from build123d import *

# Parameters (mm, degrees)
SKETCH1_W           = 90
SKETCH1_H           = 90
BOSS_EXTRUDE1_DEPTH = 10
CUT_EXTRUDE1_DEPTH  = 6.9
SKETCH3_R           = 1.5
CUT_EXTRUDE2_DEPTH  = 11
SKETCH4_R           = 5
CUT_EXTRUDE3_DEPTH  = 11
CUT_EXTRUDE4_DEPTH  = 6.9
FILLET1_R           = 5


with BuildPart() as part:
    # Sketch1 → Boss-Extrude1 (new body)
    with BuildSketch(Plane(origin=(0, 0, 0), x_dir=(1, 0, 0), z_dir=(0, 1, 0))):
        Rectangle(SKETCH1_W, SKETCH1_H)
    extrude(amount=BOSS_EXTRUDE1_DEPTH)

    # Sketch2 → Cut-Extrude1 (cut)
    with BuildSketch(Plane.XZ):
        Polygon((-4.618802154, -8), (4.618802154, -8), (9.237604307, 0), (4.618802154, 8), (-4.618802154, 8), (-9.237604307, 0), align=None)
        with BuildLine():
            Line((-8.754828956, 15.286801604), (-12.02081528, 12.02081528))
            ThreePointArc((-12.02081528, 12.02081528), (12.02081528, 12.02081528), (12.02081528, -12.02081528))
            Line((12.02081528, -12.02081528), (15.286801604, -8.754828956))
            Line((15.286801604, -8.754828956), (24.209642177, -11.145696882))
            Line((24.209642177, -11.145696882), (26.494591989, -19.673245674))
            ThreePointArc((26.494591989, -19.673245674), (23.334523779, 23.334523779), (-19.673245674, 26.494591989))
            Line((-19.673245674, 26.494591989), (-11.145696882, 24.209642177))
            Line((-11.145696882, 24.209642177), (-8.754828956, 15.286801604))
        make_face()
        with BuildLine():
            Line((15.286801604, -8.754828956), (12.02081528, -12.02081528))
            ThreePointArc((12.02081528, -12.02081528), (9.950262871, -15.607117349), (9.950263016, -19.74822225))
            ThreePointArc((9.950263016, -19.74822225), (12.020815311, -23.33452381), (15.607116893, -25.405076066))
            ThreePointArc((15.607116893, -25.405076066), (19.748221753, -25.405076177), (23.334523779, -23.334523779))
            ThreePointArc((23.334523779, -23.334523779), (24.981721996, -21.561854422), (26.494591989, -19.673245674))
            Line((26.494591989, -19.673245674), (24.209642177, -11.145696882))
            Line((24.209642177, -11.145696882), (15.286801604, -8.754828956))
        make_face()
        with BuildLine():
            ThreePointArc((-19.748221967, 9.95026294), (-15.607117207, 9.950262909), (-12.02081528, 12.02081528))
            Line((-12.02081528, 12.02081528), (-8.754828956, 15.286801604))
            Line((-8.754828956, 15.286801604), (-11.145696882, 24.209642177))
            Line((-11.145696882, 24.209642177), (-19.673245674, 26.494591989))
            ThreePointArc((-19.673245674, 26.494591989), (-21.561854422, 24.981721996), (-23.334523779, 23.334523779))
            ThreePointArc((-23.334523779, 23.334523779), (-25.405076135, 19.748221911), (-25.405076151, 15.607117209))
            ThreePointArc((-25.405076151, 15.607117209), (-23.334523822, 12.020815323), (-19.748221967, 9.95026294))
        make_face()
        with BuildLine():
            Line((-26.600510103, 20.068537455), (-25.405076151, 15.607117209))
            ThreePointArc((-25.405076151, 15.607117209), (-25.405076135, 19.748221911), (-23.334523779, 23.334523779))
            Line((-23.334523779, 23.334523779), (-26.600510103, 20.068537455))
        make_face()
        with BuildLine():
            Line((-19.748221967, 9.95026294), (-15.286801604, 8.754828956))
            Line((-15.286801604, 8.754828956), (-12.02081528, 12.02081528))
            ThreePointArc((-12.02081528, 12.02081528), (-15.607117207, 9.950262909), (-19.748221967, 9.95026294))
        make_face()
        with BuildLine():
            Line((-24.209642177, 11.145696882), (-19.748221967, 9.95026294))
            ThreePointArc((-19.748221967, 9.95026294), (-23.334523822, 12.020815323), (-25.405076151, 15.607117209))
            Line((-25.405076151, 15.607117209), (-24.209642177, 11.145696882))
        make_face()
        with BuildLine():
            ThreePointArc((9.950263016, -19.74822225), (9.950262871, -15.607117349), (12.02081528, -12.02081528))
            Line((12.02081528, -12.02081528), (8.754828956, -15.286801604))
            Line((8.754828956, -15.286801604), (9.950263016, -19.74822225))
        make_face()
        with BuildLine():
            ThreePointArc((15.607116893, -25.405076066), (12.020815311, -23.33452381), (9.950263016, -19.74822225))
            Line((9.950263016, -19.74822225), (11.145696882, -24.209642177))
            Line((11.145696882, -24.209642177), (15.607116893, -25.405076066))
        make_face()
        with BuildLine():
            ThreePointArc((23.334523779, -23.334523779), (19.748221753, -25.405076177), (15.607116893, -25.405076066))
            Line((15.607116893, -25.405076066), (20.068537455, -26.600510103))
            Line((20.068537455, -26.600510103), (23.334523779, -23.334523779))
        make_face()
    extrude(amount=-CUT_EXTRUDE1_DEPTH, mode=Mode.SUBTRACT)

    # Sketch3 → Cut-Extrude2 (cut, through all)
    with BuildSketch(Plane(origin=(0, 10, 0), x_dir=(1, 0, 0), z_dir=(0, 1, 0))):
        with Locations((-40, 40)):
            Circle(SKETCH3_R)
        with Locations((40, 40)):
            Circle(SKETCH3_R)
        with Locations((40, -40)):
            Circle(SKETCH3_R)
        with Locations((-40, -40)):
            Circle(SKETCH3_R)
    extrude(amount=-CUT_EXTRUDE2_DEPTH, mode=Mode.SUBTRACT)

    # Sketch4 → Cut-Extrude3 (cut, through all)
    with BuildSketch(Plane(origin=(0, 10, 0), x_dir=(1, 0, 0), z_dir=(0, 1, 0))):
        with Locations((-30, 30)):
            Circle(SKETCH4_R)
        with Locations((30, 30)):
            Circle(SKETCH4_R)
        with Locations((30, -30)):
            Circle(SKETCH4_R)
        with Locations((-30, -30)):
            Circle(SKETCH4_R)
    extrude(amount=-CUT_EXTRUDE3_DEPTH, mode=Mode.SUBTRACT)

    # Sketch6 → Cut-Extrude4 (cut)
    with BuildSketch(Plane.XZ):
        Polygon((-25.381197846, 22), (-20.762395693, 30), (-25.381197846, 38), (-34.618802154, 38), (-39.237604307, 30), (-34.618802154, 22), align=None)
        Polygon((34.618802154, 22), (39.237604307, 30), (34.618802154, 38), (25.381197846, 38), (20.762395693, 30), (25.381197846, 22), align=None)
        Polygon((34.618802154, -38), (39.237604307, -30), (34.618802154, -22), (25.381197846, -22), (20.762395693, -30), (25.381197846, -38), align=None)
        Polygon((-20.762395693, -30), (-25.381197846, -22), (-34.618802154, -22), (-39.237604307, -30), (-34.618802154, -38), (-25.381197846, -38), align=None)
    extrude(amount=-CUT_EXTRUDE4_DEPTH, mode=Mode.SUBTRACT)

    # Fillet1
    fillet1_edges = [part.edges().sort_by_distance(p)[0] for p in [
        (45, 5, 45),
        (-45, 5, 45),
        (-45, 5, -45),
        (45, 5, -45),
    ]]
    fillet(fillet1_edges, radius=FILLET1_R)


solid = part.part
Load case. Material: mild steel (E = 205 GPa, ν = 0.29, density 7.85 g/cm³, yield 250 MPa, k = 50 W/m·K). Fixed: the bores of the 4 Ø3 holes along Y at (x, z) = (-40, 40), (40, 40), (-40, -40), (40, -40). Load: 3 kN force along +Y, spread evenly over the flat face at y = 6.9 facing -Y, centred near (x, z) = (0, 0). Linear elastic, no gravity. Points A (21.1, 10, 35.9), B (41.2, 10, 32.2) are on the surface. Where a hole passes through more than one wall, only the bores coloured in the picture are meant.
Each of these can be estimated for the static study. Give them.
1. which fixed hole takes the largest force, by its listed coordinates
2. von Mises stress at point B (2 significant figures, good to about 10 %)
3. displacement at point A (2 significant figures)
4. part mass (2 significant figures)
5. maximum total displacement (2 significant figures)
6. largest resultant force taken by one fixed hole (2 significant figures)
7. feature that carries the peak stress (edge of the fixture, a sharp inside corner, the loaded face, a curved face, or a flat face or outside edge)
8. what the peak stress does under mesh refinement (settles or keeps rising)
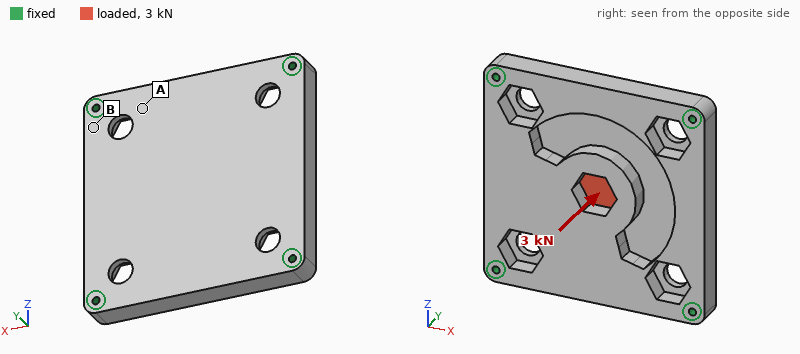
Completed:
(40, 40)
37 MPa
11 µm
480 g
48 µm
960 N
edge of the fixture
keeps rising
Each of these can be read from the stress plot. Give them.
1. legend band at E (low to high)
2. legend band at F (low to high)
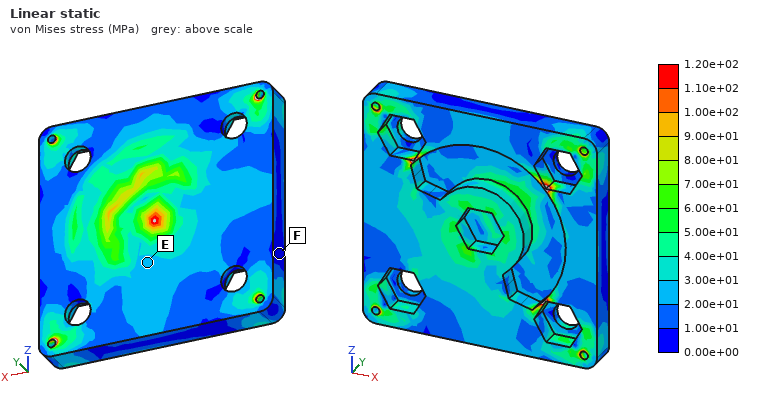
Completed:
2.00e+01 to 3.00e+01 MPa
0.00e+00 to 1.00e+01 MPa
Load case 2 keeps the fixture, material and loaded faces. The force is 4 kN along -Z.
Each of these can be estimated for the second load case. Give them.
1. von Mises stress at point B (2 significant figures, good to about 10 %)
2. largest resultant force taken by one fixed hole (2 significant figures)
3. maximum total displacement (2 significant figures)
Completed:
11 MPa
1.2 kN
5.4 µm
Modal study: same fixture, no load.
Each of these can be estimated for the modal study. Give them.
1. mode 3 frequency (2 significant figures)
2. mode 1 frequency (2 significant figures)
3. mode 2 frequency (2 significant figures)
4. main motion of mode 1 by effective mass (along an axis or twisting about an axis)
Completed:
6700 Hz
3700 Hz
6700 Hz
along Y
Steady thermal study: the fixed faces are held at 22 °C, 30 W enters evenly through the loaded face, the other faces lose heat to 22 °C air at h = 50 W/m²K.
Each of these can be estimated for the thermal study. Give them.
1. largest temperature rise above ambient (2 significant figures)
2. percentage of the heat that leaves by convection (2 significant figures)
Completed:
53 K
47 %
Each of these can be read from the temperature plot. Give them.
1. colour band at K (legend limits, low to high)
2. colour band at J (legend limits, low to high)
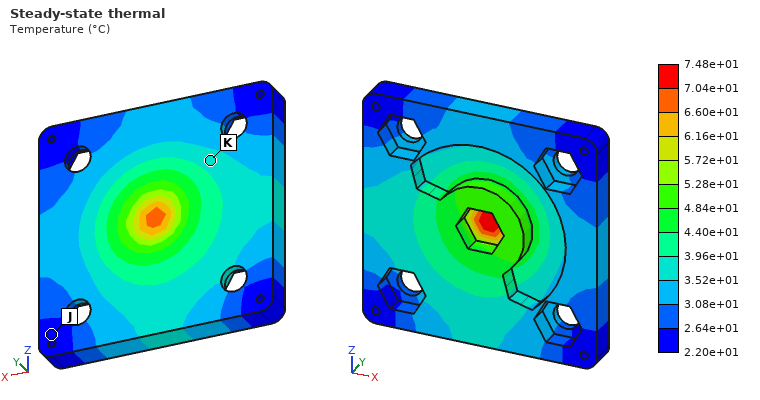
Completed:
3.52e+01 to 3.96e+01 °C
2.20e+01 to 2.64e+01 °C
